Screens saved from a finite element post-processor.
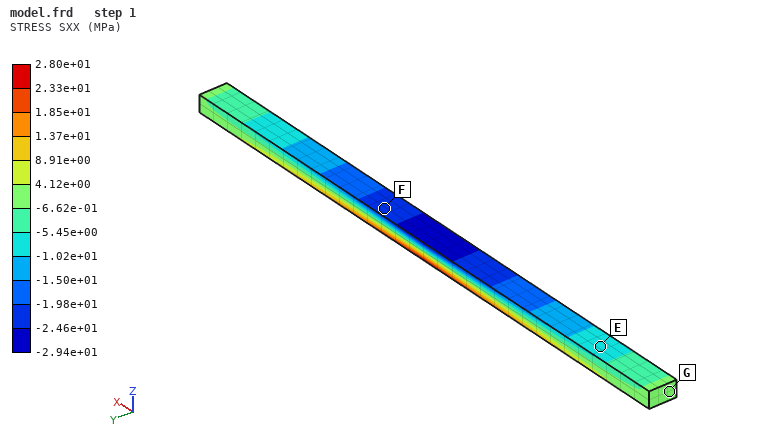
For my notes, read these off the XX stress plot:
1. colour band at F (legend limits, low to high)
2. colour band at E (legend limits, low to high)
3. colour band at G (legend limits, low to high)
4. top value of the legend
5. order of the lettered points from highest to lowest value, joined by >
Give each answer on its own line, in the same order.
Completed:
-2.46e+01 to -1.98e+01 MPa
-1.02e+01 to -5.45e+00 MPa
-6.62e-01 to 4.12e+00 MPa
2.80e+01 MPa
G > E > F
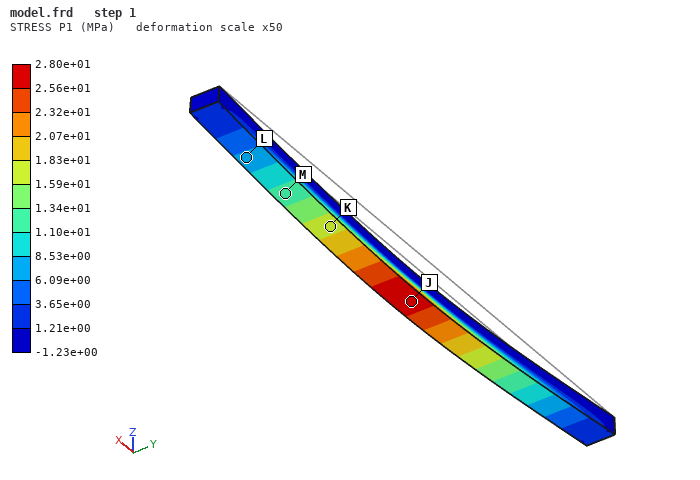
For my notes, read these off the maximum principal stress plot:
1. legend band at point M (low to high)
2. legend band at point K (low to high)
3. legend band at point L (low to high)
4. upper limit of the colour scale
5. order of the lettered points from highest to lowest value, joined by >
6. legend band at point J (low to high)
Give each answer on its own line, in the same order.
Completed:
1.10e+01 to 1.34e+01 MPa
1.59e+01 to 1.83e+01 MPa
6.09e+00 to 8.53e+00 MPa
2.80e+01 MPa
J > K > M > L
2.56e+01 to 2.80e+01 MPa
